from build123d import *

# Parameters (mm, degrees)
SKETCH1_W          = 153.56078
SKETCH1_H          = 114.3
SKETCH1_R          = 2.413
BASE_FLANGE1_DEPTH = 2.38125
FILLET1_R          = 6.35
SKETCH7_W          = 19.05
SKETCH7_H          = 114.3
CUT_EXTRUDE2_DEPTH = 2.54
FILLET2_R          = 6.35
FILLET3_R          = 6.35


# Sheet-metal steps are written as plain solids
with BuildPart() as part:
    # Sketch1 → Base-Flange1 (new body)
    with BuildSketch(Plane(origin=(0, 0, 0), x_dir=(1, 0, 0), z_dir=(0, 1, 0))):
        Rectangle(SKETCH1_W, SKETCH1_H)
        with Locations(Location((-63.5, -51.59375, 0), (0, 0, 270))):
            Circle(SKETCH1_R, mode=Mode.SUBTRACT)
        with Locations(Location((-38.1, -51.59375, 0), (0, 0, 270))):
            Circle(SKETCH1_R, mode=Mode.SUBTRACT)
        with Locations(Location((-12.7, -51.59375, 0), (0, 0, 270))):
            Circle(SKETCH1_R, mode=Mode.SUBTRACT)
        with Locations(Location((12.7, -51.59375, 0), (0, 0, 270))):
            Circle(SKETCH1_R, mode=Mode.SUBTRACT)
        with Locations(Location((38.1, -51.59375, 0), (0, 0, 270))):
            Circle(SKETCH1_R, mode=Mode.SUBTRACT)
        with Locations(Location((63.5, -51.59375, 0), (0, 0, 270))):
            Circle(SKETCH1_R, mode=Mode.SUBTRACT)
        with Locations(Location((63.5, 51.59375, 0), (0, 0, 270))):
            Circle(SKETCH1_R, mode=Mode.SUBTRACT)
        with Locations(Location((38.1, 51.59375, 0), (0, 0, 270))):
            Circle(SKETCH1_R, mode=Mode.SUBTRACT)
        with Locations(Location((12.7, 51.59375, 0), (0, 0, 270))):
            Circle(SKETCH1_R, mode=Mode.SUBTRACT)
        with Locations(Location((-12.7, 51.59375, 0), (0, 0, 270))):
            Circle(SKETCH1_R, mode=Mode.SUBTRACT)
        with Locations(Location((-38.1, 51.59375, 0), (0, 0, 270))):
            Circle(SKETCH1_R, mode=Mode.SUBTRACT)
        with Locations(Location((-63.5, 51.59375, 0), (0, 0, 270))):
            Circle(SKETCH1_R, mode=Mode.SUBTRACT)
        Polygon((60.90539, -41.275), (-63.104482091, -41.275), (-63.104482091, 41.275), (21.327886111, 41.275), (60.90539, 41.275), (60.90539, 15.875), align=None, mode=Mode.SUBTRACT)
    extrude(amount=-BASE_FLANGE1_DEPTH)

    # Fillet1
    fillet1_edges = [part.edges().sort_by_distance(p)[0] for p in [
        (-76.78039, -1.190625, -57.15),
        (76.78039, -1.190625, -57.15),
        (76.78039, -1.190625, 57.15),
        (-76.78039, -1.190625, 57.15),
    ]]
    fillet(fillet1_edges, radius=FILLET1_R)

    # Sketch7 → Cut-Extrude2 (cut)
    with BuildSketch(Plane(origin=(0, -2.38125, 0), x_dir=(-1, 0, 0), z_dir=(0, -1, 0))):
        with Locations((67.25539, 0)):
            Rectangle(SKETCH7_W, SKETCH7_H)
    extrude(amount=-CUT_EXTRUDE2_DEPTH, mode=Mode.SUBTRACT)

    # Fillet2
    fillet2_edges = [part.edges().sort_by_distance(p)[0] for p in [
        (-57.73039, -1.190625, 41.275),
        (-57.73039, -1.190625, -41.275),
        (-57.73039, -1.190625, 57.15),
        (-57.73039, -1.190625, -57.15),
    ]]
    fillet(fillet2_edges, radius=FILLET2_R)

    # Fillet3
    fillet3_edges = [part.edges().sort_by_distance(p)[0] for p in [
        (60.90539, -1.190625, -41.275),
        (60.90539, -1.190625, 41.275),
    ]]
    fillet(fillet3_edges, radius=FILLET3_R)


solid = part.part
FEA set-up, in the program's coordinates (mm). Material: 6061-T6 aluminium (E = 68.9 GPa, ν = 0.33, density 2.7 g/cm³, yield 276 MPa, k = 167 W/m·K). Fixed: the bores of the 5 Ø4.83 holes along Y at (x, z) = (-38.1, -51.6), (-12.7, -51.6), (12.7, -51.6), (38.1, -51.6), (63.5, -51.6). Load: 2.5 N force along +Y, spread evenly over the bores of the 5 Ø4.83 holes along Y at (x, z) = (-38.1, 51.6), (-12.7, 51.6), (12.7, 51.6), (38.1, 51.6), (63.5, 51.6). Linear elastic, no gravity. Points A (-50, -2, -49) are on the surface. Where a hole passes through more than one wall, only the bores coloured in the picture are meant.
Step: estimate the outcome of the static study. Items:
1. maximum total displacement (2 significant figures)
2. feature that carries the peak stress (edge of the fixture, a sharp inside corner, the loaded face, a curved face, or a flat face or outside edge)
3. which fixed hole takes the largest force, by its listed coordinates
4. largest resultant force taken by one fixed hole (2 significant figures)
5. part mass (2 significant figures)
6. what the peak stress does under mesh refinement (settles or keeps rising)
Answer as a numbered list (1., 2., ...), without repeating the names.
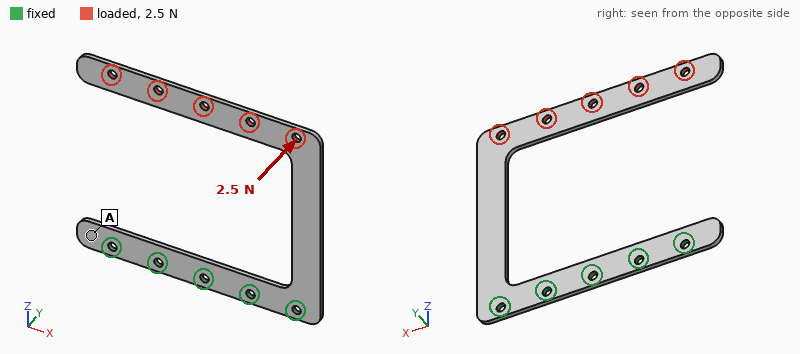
1. 2.0 mm
2. edge of the fixture
3. (63.5, -51.6)
4. 2.5 N
5. 34 g
6. keeps rising
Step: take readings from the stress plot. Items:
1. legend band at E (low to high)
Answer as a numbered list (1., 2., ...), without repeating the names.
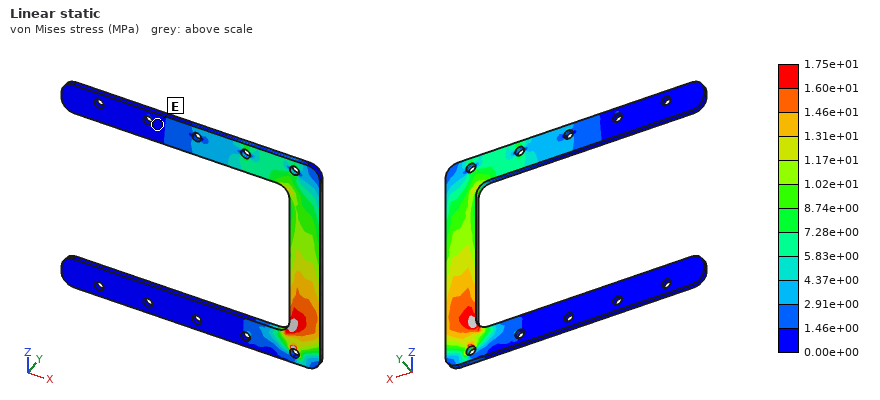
1. 0.00e+00 to 1.46e+00 MPa
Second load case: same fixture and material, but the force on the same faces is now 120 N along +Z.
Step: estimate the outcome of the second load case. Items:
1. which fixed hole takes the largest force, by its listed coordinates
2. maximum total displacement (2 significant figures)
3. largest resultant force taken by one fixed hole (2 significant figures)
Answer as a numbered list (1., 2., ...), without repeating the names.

1. (38.1, -51.6)
2. 2.0 mm
3. 240 N
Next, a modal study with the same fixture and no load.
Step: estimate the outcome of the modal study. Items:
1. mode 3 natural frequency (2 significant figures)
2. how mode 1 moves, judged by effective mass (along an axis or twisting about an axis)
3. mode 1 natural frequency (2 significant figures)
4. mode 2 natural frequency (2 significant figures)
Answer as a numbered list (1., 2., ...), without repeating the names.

1. 350 Hz
2. along Y
3. 58 Hz
4. 160 Hz
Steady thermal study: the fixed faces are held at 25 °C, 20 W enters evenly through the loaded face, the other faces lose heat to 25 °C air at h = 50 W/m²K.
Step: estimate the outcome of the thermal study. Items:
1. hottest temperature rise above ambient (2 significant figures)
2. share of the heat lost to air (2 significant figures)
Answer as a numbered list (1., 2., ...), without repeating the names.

1. 74 K
2. 90 %
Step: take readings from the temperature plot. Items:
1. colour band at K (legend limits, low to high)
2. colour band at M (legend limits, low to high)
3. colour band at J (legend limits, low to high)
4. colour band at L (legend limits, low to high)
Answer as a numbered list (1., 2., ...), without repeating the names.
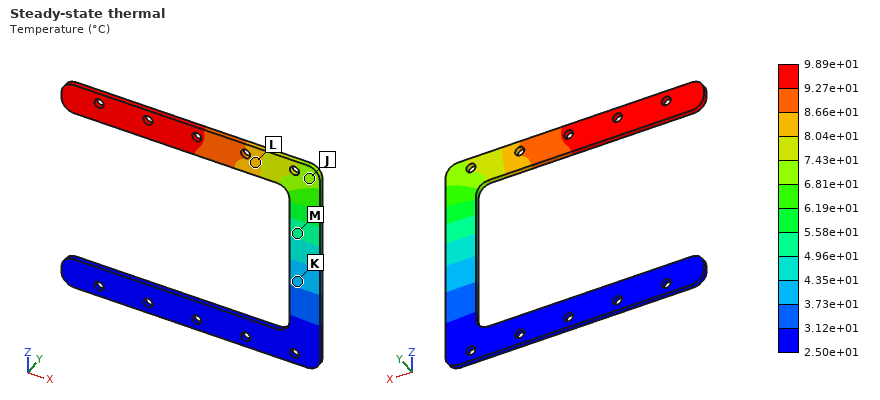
1. 3.73e+01 to 4.35e+01 °C
2. 4.96e+01 to 5.58e+01 °C
3. 6.81e+01 to 7.43e+01 °C
4. 8.04e+01 to 8.66e+01 °C
